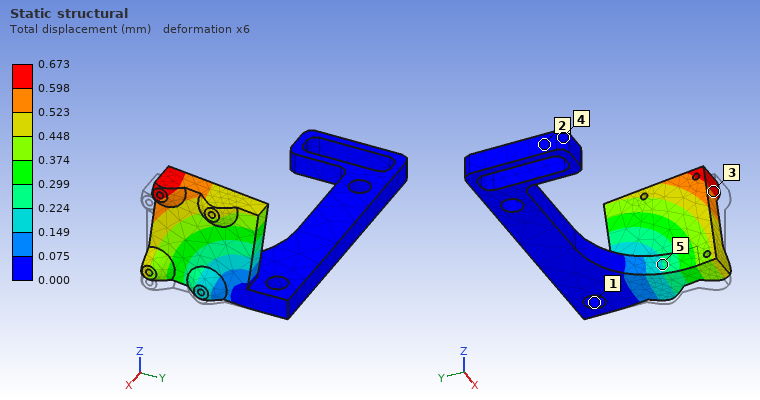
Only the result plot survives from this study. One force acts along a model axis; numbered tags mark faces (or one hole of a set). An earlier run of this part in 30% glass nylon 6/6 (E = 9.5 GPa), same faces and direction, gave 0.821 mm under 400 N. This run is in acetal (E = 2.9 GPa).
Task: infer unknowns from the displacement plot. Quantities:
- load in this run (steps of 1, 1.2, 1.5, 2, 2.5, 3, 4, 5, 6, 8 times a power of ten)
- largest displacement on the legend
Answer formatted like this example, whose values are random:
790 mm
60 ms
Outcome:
100 N
0.673 mm
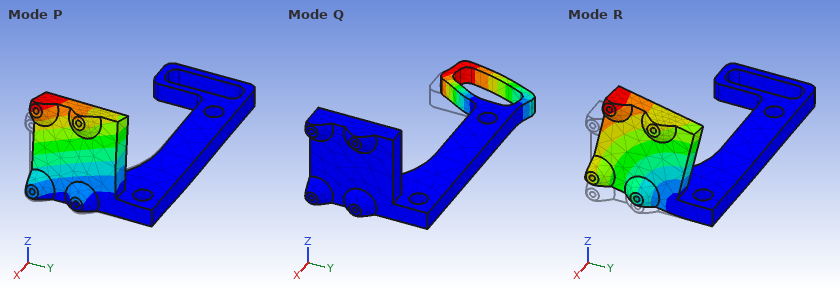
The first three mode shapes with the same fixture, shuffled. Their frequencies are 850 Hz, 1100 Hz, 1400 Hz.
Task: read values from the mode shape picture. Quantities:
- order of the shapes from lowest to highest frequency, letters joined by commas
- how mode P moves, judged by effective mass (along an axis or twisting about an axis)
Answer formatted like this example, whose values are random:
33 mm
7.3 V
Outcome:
R, P, Q
along X
